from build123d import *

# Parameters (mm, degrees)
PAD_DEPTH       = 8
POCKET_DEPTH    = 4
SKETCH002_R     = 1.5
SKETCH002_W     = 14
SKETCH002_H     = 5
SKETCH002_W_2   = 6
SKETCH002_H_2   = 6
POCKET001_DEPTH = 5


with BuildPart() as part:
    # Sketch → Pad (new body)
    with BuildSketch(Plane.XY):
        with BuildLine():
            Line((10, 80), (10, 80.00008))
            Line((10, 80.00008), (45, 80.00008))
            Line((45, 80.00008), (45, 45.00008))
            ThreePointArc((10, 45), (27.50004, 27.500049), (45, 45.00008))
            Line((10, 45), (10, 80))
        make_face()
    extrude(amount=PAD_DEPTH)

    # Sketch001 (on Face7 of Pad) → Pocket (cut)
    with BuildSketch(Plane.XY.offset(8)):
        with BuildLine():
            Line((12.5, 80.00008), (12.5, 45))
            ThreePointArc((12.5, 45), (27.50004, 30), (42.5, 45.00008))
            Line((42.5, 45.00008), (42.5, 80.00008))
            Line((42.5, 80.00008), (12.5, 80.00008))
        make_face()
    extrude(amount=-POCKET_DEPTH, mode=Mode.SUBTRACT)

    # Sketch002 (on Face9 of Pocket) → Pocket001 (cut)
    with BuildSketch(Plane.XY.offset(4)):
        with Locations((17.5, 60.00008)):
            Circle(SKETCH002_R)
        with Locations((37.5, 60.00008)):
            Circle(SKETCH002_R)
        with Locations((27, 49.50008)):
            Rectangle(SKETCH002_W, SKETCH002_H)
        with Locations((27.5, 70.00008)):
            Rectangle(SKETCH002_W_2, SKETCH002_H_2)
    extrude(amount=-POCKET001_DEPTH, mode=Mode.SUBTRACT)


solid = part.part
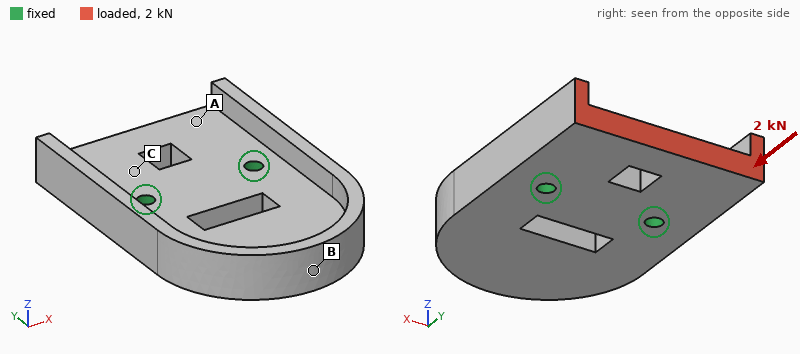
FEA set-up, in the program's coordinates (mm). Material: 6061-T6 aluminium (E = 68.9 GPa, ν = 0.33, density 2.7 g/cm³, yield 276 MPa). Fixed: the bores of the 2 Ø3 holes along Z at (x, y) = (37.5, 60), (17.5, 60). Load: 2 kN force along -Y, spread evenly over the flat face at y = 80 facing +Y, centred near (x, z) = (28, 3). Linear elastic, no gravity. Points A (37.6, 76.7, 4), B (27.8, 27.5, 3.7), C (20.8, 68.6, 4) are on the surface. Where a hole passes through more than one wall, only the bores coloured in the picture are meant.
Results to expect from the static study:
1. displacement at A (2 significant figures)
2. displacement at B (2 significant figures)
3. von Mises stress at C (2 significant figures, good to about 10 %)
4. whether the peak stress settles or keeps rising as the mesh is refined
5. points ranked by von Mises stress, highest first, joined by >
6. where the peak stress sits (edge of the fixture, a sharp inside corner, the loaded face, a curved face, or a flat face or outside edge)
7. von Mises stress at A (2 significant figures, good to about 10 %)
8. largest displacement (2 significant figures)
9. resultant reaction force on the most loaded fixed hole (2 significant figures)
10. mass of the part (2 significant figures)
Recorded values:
6.5 µm
11 µm
19 MPa
keeps rising
C > A > B
edge of the fixture
13 MPa
11 µm
1.0 kN
20 g
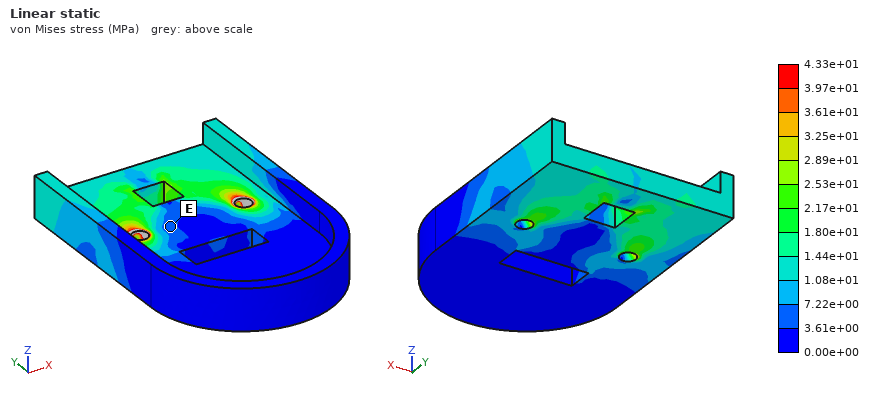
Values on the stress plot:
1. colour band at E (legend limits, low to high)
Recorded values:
3.61e+00 to 7.22e+00 MPa
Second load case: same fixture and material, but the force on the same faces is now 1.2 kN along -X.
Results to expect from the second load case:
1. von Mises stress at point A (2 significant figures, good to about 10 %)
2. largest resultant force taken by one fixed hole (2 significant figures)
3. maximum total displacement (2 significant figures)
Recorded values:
21 MPa
1.2 kN
34 µm
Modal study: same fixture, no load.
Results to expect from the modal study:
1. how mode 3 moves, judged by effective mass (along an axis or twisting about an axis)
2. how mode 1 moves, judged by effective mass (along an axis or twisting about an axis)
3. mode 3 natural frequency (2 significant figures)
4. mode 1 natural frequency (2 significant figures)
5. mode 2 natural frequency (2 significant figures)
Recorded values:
along Z
along Z
8900 Hz
3500 Hz
8000 Hz
